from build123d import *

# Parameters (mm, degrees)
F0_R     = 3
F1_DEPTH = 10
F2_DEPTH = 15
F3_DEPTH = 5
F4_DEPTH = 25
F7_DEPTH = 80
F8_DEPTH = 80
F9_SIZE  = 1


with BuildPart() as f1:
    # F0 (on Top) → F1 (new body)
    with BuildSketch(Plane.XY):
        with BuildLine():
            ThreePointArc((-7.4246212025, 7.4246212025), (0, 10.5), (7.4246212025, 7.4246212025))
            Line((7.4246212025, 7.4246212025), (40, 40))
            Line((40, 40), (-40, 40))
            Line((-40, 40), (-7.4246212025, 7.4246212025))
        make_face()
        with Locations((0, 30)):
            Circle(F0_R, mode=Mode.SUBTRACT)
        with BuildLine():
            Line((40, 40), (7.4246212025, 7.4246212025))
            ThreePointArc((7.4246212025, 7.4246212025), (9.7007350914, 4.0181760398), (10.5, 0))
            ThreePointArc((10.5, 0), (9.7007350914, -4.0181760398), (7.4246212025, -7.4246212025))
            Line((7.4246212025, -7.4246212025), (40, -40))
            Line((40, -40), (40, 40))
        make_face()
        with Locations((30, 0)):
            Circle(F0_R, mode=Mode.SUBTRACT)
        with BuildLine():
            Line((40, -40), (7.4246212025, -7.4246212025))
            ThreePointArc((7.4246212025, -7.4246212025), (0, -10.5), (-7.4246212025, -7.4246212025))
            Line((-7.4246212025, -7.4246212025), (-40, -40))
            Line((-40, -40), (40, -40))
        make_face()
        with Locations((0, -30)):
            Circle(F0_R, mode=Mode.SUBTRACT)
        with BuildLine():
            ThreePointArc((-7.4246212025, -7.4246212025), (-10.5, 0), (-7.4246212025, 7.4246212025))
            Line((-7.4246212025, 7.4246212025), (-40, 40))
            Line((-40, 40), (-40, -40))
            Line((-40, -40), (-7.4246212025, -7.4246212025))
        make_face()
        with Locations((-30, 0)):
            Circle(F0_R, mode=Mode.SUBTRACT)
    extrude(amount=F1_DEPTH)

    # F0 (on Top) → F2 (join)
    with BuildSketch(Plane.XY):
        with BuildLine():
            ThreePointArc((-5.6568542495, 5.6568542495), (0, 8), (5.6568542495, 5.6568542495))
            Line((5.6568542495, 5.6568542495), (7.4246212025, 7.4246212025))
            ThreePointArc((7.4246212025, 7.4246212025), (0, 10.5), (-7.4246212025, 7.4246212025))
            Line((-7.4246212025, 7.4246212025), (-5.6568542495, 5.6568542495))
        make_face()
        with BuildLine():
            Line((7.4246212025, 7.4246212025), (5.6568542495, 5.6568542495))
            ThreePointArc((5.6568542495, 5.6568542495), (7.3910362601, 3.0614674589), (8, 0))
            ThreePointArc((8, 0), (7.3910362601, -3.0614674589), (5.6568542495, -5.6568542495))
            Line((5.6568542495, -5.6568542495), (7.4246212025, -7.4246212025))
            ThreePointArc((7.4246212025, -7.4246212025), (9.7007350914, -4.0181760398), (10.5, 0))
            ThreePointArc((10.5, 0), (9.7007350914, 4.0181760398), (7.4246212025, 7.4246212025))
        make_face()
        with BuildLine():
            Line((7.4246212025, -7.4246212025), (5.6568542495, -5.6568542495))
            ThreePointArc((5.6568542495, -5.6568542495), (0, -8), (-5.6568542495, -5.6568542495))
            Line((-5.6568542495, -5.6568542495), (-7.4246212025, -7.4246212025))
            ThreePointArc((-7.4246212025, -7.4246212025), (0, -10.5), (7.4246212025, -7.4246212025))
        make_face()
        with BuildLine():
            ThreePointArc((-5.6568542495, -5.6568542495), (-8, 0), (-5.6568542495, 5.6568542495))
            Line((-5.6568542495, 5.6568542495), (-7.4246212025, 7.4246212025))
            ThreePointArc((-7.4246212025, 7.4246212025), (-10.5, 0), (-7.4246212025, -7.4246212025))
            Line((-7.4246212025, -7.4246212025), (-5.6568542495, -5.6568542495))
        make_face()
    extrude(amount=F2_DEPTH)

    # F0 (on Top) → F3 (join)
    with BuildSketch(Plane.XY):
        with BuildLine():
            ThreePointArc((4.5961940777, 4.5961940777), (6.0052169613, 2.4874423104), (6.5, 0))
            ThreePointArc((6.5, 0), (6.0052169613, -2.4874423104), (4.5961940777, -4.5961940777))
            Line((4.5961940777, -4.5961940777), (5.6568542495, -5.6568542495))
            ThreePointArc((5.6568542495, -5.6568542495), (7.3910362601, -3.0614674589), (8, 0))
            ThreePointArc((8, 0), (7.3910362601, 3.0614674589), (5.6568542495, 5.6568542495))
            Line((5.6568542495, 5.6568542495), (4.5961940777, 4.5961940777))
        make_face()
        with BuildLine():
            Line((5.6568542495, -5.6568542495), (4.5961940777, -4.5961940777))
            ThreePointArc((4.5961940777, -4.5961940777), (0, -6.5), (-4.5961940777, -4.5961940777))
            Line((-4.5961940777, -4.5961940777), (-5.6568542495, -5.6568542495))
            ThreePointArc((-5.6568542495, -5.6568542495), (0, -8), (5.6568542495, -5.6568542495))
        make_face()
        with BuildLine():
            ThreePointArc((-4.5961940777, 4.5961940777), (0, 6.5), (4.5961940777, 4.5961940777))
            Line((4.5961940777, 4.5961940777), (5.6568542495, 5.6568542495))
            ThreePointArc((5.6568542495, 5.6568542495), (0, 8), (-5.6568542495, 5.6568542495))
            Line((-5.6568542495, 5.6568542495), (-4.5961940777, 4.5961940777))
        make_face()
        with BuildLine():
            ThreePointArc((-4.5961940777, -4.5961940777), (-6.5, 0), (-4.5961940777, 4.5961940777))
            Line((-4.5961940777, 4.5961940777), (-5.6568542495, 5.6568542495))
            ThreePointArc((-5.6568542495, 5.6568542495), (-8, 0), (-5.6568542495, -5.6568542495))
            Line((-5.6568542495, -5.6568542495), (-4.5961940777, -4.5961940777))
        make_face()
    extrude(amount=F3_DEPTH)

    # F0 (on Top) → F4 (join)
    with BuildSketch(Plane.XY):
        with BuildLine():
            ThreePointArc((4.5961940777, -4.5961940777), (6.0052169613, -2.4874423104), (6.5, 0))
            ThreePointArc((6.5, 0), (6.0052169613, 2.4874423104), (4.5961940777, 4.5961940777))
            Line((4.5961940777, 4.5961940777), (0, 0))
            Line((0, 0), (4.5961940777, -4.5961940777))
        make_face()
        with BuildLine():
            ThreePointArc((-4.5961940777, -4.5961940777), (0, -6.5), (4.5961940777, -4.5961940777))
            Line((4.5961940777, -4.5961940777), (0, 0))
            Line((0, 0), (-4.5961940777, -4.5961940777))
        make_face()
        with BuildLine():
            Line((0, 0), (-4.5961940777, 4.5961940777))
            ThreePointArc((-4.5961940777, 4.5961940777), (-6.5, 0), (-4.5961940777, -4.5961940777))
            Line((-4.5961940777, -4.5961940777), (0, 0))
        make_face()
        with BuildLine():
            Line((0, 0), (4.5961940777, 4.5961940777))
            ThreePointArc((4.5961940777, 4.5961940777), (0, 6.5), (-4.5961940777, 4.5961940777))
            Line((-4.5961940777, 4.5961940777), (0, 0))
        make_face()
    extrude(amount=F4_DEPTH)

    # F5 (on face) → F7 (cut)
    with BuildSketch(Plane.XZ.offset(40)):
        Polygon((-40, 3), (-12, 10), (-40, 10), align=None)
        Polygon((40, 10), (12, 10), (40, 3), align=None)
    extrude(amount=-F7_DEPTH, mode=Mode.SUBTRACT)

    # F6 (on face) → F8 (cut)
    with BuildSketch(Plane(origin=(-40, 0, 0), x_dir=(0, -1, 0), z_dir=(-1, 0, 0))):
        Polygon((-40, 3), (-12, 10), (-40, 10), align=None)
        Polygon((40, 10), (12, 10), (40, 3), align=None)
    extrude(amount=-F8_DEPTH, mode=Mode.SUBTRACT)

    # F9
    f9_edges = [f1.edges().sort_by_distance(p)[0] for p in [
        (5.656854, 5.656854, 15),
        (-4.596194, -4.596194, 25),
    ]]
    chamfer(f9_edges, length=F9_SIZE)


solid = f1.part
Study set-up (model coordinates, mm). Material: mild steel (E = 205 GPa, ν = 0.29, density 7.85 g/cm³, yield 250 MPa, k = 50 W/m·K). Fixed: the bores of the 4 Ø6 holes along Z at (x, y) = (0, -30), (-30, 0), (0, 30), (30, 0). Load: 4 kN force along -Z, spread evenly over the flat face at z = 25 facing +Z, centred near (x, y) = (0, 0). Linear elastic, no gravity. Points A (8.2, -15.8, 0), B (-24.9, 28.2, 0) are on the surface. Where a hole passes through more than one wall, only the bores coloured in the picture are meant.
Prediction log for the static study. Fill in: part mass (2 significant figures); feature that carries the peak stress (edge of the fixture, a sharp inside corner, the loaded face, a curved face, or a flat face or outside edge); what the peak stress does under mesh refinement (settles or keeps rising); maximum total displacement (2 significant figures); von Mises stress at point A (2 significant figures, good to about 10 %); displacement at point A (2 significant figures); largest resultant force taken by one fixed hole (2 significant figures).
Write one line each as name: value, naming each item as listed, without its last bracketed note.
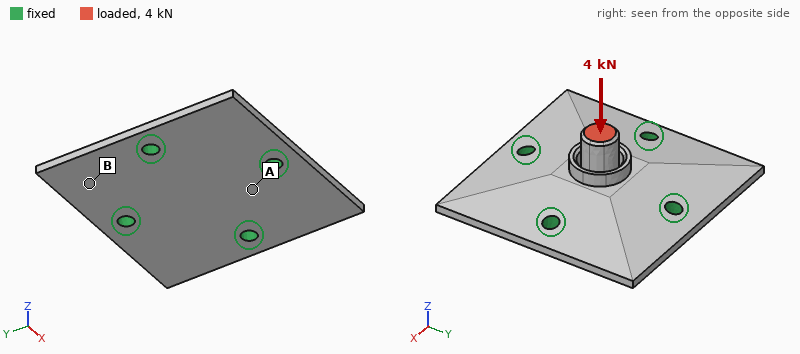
part mass: 330 g
feature that carries the peak stress: edge of the fixture
what the peak stress does under mesh refinement: keeps rising
maximum total displacement: 13 µm
von Mises stress at point A: 16 MPa
displacement at point A: 4.3 µm
largest resultant force taken by one fixed hole: 1.2 kN
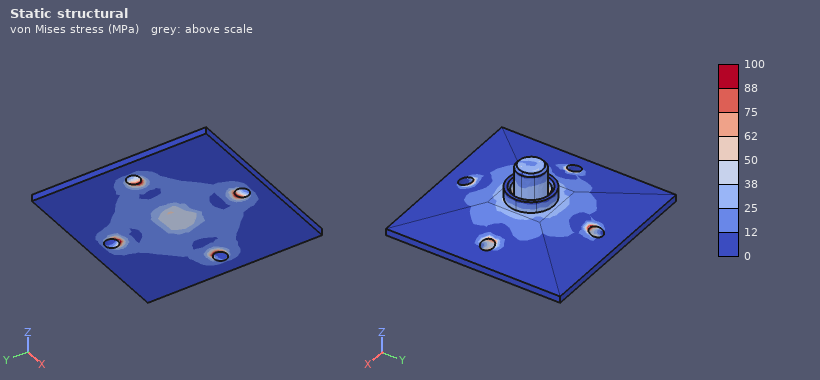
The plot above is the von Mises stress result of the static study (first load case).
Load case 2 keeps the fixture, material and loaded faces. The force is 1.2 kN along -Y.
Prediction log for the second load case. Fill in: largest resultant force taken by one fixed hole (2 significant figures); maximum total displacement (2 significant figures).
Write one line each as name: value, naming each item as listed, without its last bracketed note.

largest resultant force taken by one fixed hole: 710 N
maximum total displacement: 28 µm
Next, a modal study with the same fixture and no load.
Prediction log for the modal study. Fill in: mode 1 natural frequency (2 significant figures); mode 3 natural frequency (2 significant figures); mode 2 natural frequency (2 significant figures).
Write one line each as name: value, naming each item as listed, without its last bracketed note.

mode 1 natural frequency: 6900 Hz
mode 3 natural frequency: 7200 Hz
mode 2 natural frequency: 7200 Hz
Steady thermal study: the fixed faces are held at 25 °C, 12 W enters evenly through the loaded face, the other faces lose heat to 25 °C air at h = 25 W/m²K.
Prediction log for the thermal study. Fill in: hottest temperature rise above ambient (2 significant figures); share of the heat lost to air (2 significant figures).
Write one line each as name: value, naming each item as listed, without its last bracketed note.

hottest temperature rise above ambient: 49 K
share of the heat lost to air: 13 %
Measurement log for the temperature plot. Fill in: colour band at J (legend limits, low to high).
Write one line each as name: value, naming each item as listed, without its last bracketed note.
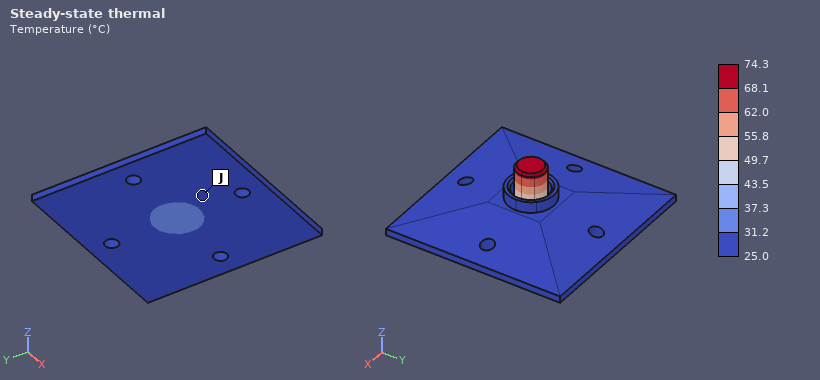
colour band at J: 25.0 to 31.2 °C
